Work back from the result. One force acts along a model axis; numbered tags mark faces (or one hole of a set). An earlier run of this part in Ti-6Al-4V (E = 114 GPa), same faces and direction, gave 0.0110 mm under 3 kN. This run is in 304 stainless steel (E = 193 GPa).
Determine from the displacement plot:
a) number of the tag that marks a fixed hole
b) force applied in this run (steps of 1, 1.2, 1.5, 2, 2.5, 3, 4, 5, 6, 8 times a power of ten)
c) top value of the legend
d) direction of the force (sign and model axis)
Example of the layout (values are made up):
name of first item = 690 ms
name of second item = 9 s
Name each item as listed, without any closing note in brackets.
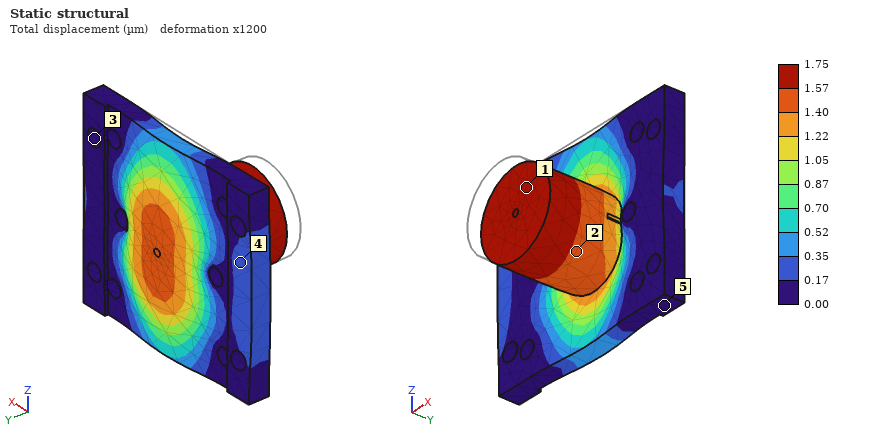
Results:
number of the tag that marks a fixed hole = 3
force applied in this run = 800 N
top value of the legend = 1.75 µm
direction of the force = +Y
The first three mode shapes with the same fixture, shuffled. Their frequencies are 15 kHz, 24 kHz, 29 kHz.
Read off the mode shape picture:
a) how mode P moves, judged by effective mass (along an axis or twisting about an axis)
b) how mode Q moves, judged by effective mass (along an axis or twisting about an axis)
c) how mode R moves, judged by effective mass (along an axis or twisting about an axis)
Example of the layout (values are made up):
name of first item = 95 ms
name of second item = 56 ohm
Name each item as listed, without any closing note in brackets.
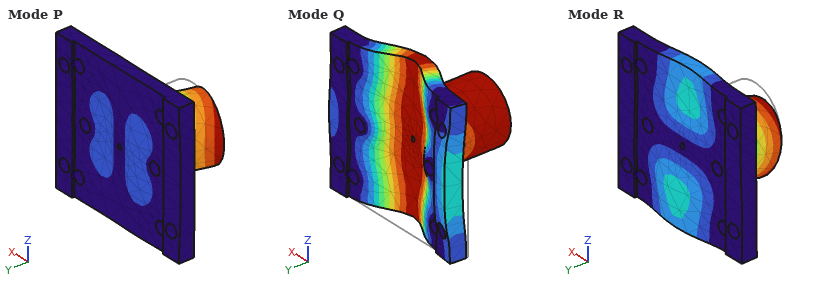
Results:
how mode P moves, judged by effective mass = along X
how mode Q moves, judged by effective mass = along Y
how mode R moves, judged by effective mass = along Z
